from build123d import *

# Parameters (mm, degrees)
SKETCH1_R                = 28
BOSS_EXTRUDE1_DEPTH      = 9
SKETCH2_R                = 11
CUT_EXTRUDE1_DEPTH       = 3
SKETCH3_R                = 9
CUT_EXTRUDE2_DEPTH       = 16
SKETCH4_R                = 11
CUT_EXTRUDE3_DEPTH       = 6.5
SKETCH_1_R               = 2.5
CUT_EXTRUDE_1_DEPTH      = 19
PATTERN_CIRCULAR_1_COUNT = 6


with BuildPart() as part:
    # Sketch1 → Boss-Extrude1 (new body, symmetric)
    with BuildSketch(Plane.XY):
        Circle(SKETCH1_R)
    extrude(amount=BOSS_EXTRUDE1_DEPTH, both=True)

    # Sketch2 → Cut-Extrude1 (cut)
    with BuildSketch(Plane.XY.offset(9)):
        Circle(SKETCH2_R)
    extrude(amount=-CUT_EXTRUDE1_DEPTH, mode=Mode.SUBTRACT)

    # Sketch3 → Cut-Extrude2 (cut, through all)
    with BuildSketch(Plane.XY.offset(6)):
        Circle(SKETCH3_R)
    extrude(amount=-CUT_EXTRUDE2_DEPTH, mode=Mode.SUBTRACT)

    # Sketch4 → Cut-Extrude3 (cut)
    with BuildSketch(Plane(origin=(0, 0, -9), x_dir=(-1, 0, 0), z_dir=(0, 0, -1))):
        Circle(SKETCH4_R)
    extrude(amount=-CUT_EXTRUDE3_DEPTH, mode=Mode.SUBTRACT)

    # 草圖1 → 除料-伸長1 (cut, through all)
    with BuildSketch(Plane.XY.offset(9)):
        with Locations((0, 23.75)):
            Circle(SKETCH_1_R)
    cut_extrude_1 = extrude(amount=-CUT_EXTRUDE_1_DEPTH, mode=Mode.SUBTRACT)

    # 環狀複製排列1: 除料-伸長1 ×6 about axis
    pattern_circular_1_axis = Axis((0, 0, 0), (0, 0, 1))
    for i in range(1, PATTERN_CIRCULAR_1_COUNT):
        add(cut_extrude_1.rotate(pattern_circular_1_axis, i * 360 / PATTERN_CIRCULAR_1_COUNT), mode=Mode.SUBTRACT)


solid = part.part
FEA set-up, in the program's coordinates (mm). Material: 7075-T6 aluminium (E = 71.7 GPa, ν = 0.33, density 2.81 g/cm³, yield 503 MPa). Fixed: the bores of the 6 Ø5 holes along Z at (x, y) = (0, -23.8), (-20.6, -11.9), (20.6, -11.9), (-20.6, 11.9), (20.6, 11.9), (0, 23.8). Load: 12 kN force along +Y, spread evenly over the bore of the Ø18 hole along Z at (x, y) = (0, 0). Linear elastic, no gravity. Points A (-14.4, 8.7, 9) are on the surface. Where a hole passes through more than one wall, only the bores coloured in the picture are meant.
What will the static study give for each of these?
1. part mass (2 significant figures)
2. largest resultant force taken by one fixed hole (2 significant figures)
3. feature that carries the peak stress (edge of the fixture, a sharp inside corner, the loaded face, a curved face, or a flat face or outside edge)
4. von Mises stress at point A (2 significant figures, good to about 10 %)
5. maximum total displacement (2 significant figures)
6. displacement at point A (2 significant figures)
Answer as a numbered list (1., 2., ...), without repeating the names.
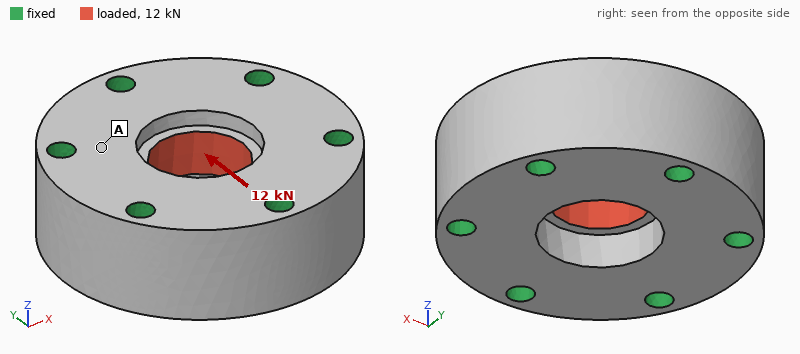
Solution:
1. 100 g
2. 3.0 kN
3. a sharp inside corner
4. 8.4 MPa
5. 4.1 µm
6. 1.1 µm
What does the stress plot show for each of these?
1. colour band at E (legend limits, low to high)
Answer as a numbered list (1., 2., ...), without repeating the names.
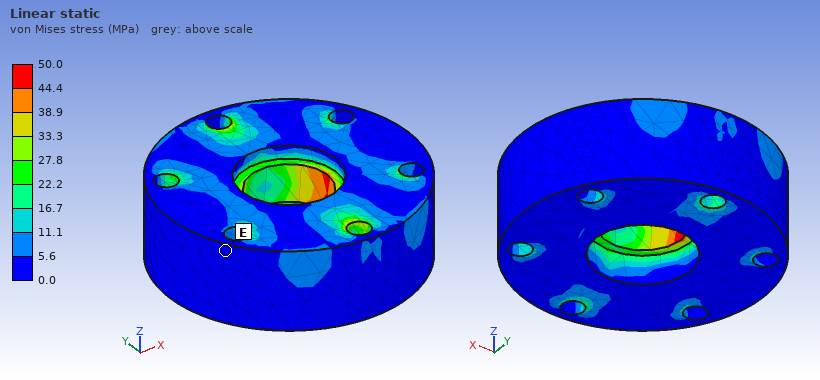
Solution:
1. 0.0 to 5.6 MPa
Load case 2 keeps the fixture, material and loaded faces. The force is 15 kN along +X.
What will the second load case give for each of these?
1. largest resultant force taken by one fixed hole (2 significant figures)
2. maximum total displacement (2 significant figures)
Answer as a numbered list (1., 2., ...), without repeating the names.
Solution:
1. 3.3 kN
2. 5.2 µm
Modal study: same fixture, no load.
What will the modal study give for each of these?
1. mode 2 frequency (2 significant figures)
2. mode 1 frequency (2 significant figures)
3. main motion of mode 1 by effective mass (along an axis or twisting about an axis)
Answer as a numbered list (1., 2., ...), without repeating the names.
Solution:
1. 54 kHz
2. 44 kHz
3. along Z
